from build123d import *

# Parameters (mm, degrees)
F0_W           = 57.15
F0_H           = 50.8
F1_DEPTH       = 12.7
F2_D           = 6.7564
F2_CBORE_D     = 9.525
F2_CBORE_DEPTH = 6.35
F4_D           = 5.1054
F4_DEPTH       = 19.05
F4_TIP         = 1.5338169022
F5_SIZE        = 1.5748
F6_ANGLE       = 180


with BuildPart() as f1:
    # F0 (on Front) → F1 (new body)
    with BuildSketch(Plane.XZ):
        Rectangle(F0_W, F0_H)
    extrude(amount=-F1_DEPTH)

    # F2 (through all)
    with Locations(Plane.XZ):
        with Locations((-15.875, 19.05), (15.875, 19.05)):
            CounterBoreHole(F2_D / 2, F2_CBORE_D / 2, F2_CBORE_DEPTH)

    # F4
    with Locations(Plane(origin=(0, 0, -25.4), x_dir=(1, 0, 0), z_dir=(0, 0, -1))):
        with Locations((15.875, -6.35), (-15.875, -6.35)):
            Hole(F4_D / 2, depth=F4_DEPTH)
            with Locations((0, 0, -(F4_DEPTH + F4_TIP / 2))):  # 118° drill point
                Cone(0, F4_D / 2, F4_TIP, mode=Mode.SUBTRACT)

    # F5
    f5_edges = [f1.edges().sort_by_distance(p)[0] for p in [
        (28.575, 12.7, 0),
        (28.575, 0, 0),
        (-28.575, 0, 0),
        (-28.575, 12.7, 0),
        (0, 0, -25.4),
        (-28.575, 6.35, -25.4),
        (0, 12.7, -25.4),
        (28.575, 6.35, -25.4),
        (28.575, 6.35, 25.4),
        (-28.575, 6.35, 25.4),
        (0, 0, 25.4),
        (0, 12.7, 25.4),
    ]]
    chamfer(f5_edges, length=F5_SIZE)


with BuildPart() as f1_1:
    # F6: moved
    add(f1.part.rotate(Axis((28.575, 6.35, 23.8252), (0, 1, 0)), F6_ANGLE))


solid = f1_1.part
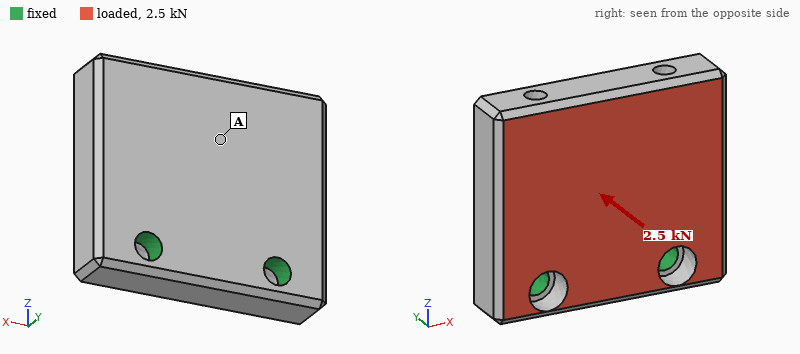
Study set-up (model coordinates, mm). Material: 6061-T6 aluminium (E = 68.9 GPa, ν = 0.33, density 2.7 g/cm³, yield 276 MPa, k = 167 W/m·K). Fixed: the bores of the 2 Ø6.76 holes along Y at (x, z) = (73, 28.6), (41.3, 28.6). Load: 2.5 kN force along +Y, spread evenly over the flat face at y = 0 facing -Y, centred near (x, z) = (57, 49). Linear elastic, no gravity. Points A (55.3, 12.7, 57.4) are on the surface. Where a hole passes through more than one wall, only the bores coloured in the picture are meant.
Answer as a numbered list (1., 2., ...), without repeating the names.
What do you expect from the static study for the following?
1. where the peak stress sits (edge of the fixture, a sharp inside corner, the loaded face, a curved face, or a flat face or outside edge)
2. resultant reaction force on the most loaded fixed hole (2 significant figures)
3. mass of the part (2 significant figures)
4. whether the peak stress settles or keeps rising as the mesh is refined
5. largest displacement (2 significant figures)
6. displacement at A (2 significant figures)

1. edge of the fixture
2. 1.3 kN
3. 92 g
4. keeps rising
5. 0.10 mm
6. 0.063 mm
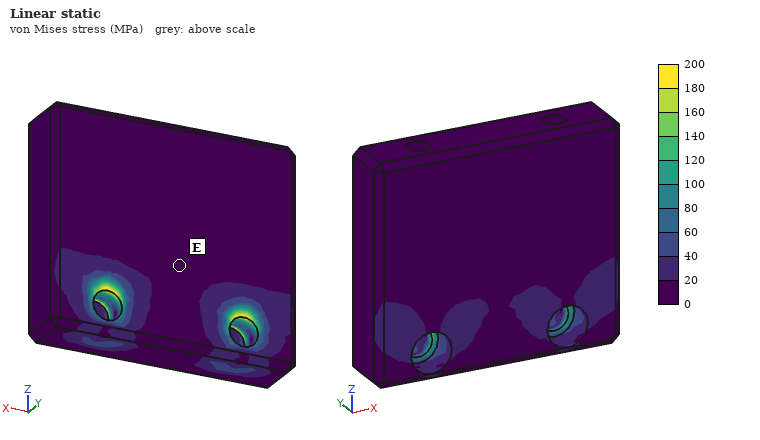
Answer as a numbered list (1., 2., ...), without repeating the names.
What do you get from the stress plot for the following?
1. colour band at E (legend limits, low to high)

1. 0 to 20 MPa
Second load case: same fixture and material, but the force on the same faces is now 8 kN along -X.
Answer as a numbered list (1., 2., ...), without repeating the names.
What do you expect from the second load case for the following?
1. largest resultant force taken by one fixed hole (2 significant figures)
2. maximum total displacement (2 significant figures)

1. 6.3 kN
2. 42 µm
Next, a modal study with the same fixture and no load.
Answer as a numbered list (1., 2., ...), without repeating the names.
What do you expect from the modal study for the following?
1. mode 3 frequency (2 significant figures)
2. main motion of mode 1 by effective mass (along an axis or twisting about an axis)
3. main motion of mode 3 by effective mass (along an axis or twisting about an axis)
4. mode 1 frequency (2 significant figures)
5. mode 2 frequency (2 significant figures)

1. 10 kHz
2. along Y
3. along X
4. 3200 Hz
5. 7700 Hz
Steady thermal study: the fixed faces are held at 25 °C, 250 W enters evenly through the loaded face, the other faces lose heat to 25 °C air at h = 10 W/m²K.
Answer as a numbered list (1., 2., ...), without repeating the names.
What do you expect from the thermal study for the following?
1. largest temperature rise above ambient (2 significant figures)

1. 58 K
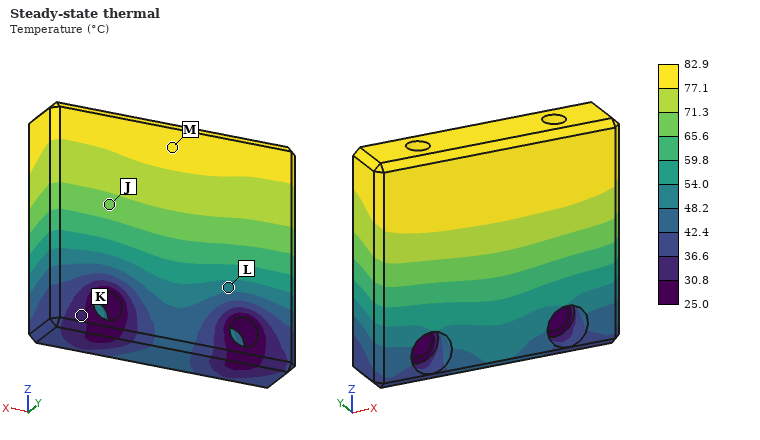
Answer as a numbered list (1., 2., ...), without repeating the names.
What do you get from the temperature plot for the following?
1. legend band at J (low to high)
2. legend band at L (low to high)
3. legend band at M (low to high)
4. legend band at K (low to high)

1. 65.6 to 71.3 °C
2. 48.2 to 54.0 °C
3. 77.1 to 82.9 °C
4. 30.8 to 36.6 °C
